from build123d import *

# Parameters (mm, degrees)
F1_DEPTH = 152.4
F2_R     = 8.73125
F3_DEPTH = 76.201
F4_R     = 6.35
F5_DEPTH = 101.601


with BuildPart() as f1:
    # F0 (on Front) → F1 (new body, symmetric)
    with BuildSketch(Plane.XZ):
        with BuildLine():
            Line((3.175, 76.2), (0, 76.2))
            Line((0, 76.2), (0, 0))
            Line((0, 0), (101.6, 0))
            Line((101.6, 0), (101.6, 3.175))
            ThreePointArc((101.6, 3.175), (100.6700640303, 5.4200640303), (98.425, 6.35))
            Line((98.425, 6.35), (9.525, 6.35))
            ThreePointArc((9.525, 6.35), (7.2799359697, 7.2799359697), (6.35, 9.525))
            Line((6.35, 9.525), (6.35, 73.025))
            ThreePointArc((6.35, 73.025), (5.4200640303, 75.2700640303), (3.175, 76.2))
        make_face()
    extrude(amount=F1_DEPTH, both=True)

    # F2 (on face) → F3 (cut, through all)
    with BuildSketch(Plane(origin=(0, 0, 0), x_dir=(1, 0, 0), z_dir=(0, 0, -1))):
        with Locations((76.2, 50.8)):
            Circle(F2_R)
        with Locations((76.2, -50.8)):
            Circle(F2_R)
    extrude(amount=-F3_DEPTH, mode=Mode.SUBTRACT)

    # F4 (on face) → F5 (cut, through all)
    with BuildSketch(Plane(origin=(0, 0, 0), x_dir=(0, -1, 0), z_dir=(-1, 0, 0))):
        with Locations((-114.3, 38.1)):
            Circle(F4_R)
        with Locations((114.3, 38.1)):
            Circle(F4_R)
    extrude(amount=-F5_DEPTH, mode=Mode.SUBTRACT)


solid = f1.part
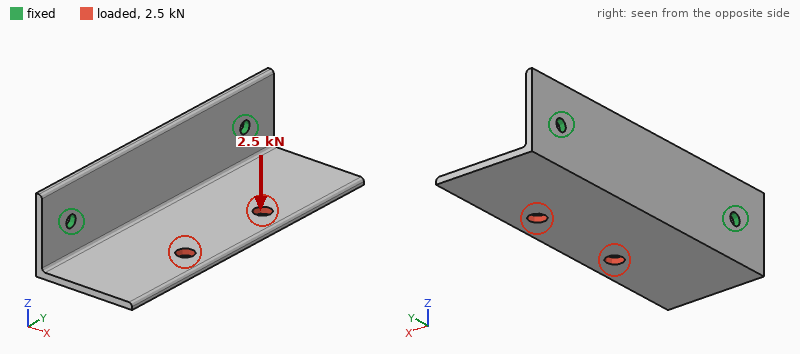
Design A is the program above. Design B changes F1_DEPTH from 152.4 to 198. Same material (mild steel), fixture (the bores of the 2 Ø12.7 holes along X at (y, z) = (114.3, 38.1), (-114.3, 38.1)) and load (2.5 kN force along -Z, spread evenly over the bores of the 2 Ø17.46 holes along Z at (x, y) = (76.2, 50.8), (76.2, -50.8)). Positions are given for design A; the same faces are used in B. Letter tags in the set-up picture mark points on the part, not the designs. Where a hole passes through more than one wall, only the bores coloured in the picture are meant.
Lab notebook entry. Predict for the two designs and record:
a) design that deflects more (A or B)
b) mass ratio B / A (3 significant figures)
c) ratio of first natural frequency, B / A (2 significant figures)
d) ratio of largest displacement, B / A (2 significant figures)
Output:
A
1.30
0.97
0.90
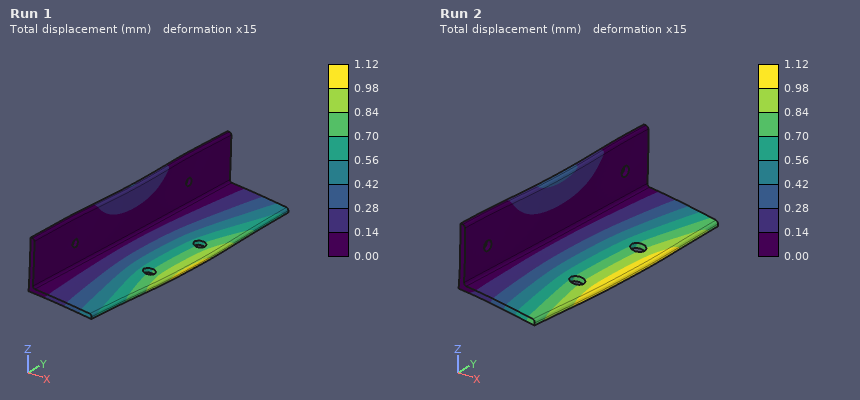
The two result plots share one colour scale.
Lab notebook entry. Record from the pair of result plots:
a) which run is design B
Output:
Run 1
